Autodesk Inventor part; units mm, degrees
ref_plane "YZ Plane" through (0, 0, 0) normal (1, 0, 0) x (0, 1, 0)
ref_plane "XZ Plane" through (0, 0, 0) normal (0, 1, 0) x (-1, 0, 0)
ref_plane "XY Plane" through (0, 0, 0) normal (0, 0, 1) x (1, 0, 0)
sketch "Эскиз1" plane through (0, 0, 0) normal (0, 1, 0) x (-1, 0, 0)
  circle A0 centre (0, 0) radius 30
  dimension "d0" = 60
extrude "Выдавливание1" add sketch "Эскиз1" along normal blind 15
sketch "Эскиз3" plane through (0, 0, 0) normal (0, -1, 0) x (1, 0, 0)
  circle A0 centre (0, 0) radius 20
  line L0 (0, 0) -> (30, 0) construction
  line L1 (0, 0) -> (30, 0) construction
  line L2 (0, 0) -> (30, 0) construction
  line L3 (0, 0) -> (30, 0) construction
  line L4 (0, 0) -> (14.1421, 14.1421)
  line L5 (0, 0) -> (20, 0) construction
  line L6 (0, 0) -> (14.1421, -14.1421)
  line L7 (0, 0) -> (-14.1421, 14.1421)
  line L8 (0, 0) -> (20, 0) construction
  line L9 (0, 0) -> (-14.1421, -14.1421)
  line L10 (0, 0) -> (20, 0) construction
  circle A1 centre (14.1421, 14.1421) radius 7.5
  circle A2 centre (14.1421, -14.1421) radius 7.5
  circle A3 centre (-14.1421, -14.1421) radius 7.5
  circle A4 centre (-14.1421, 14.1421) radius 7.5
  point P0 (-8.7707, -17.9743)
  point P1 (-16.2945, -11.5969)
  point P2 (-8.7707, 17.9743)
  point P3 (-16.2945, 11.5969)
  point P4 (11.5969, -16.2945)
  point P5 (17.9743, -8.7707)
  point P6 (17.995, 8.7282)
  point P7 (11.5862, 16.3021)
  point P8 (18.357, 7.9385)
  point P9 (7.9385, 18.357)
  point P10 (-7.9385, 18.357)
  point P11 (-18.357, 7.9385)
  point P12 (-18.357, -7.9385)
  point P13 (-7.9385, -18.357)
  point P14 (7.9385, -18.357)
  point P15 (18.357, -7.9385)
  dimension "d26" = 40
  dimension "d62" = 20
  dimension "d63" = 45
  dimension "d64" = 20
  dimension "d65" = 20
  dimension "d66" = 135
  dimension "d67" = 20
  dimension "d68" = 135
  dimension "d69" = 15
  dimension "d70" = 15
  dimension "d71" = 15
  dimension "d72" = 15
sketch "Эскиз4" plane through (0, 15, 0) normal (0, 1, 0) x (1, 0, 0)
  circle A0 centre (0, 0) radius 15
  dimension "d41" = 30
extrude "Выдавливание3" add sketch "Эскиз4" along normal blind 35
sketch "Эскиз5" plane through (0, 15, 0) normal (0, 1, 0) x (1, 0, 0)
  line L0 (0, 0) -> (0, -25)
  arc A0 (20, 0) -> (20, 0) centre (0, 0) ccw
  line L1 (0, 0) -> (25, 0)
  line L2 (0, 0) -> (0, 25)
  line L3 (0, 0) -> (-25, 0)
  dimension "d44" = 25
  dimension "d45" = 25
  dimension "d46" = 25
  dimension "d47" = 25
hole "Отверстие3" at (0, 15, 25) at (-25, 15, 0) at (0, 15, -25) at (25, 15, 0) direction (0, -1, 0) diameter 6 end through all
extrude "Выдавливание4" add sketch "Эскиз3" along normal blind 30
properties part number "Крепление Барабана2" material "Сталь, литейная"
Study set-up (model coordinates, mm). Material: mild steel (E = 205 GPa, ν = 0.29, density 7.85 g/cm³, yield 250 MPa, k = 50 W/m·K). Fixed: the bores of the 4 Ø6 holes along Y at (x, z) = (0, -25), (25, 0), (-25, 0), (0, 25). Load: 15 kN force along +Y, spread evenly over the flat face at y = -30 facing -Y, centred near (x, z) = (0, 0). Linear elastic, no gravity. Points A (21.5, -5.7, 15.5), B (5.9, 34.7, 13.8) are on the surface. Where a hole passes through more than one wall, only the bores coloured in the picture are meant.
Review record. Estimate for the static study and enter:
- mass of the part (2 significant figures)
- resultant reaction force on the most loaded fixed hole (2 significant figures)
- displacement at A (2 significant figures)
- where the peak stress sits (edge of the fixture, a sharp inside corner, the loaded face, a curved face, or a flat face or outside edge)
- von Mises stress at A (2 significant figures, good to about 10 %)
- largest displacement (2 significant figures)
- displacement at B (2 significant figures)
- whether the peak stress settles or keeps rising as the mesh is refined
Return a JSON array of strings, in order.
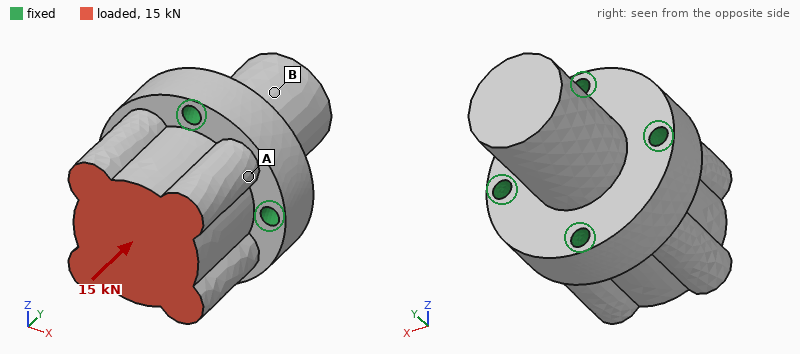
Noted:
["900 g", "3.8 kN", "1.8 µm", "edge of the fixture", "10 MPa", "2.9 µm", "1.4 µm", "keeps rising"]
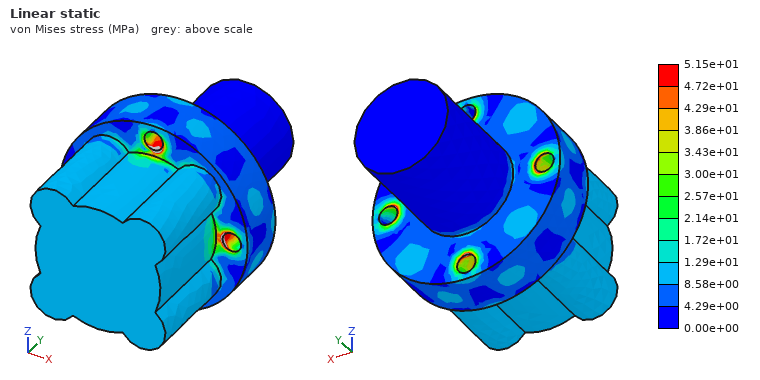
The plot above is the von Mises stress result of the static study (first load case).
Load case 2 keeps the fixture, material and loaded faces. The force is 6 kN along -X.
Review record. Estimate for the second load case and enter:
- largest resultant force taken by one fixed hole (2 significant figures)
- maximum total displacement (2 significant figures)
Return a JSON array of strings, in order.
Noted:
["4.6 kN", "7.1 µm"]
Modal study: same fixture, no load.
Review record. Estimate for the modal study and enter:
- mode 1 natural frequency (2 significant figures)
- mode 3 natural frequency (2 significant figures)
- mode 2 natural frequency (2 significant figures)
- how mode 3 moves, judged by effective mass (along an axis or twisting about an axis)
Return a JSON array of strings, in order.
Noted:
["9300 Hz", "13 kHz", "9300 Hz", "along X"]
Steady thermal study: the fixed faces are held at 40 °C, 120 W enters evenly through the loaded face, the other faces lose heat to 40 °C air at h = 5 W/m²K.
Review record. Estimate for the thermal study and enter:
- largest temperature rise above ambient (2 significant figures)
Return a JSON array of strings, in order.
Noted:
["63 K"]
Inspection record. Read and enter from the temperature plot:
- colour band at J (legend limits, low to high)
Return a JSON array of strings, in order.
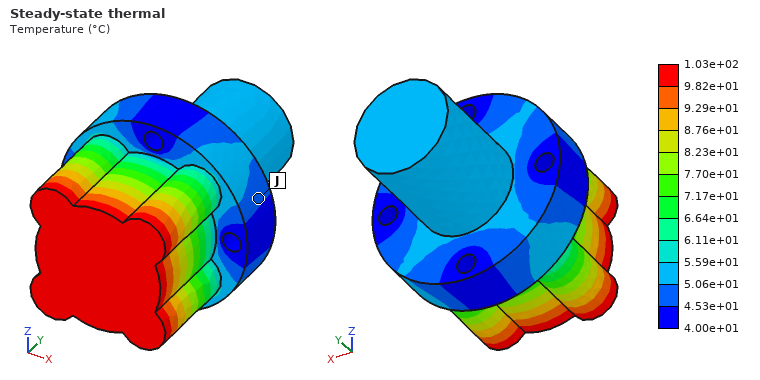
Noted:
["4.53e+01 to 5.06e+01 °C"]
